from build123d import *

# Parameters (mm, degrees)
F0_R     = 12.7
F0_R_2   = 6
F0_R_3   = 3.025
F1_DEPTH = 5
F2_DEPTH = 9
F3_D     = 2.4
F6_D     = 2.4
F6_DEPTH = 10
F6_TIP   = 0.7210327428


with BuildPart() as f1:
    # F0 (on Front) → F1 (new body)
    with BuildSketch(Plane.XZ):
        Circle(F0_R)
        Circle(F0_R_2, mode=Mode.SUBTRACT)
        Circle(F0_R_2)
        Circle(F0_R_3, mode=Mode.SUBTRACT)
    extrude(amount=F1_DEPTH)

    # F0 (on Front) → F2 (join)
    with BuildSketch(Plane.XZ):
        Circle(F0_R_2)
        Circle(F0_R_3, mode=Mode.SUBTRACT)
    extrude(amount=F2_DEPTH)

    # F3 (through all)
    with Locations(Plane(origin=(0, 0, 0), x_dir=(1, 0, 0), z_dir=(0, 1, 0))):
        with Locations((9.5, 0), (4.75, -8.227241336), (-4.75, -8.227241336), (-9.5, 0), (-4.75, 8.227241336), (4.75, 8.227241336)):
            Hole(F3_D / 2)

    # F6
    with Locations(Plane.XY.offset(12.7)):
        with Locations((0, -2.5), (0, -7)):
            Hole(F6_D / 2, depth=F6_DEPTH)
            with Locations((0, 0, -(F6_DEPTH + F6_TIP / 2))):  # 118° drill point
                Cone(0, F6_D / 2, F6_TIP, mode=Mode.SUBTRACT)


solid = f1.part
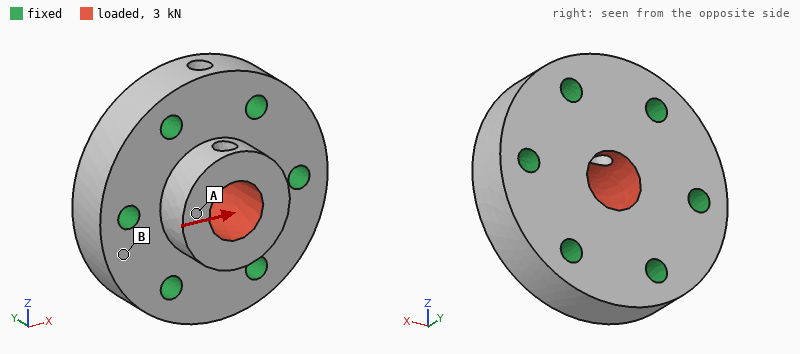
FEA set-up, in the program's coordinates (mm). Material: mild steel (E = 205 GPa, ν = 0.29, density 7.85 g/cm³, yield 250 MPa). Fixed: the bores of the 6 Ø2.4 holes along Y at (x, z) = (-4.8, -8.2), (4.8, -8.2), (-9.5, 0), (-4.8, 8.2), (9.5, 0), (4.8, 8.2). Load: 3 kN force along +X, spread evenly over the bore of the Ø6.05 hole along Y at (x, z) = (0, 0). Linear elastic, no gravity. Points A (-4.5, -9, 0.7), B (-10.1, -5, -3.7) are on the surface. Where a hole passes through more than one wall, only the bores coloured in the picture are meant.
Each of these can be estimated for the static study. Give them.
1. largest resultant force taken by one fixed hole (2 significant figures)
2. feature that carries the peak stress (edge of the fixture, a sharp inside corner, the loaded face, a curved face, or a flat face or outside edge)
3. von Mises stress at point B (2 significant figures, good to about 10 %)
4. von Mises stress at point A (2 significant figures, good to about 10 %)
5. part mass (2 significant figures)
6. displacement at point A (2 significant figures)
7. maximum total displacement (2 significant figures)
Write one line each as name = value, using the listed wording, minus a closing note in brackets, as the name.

largest resultant force taken by one fixed hole = 810 N
feature that carries the peak stress = the loaded face
von Mises stress at point B = 7.4 MPa
von Mises stress at point A = 28 MPa
part mass = 20 g
displacement at point A = 2.2 µm
maximum total displacement = 2.4 µm
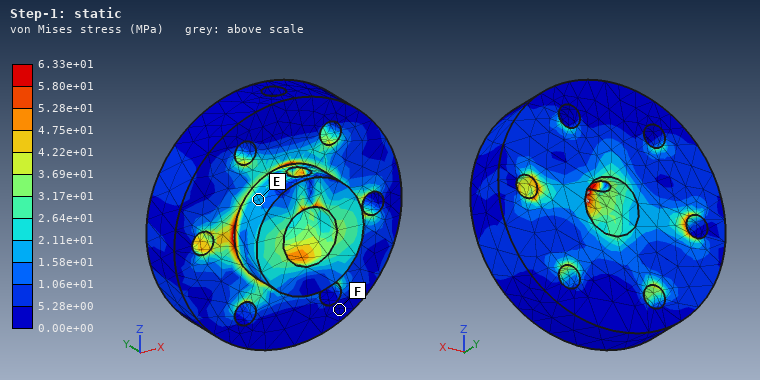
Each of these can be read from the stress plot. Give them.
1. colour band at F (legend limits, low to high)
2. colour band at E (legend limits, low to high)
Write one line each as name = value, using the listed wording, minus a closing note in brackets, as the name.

colour band at F = 0.00e+00 to 5.28e+00 MPa
colour band at E = 1.58e+01 to 2.11e+01 MPa
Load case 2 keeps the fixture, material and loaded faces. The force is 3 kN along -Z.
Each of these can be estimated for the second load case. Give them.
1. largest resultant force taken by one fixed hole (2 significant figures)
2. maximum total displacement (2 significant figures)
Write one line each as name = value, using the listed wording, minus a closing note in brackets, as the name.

largest resultant force taken by one fixed hole = 720 N
maximum total displacement = 2.2 µm
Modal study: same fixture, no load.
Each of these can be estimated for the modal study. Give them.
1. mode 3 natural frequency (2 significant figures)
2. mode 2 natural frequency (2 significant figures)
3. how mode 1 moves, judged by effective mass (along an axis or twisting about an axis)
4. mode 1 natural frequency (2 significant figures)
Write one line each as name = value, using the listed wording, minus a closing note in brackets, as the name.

mode 3 natural frequency = 96 kHz
mode 2 natural frequency = 94 kHz
how mode 1 moves, judged by effective mass = along Y
mode 1 natural frequency = 87 kHz
